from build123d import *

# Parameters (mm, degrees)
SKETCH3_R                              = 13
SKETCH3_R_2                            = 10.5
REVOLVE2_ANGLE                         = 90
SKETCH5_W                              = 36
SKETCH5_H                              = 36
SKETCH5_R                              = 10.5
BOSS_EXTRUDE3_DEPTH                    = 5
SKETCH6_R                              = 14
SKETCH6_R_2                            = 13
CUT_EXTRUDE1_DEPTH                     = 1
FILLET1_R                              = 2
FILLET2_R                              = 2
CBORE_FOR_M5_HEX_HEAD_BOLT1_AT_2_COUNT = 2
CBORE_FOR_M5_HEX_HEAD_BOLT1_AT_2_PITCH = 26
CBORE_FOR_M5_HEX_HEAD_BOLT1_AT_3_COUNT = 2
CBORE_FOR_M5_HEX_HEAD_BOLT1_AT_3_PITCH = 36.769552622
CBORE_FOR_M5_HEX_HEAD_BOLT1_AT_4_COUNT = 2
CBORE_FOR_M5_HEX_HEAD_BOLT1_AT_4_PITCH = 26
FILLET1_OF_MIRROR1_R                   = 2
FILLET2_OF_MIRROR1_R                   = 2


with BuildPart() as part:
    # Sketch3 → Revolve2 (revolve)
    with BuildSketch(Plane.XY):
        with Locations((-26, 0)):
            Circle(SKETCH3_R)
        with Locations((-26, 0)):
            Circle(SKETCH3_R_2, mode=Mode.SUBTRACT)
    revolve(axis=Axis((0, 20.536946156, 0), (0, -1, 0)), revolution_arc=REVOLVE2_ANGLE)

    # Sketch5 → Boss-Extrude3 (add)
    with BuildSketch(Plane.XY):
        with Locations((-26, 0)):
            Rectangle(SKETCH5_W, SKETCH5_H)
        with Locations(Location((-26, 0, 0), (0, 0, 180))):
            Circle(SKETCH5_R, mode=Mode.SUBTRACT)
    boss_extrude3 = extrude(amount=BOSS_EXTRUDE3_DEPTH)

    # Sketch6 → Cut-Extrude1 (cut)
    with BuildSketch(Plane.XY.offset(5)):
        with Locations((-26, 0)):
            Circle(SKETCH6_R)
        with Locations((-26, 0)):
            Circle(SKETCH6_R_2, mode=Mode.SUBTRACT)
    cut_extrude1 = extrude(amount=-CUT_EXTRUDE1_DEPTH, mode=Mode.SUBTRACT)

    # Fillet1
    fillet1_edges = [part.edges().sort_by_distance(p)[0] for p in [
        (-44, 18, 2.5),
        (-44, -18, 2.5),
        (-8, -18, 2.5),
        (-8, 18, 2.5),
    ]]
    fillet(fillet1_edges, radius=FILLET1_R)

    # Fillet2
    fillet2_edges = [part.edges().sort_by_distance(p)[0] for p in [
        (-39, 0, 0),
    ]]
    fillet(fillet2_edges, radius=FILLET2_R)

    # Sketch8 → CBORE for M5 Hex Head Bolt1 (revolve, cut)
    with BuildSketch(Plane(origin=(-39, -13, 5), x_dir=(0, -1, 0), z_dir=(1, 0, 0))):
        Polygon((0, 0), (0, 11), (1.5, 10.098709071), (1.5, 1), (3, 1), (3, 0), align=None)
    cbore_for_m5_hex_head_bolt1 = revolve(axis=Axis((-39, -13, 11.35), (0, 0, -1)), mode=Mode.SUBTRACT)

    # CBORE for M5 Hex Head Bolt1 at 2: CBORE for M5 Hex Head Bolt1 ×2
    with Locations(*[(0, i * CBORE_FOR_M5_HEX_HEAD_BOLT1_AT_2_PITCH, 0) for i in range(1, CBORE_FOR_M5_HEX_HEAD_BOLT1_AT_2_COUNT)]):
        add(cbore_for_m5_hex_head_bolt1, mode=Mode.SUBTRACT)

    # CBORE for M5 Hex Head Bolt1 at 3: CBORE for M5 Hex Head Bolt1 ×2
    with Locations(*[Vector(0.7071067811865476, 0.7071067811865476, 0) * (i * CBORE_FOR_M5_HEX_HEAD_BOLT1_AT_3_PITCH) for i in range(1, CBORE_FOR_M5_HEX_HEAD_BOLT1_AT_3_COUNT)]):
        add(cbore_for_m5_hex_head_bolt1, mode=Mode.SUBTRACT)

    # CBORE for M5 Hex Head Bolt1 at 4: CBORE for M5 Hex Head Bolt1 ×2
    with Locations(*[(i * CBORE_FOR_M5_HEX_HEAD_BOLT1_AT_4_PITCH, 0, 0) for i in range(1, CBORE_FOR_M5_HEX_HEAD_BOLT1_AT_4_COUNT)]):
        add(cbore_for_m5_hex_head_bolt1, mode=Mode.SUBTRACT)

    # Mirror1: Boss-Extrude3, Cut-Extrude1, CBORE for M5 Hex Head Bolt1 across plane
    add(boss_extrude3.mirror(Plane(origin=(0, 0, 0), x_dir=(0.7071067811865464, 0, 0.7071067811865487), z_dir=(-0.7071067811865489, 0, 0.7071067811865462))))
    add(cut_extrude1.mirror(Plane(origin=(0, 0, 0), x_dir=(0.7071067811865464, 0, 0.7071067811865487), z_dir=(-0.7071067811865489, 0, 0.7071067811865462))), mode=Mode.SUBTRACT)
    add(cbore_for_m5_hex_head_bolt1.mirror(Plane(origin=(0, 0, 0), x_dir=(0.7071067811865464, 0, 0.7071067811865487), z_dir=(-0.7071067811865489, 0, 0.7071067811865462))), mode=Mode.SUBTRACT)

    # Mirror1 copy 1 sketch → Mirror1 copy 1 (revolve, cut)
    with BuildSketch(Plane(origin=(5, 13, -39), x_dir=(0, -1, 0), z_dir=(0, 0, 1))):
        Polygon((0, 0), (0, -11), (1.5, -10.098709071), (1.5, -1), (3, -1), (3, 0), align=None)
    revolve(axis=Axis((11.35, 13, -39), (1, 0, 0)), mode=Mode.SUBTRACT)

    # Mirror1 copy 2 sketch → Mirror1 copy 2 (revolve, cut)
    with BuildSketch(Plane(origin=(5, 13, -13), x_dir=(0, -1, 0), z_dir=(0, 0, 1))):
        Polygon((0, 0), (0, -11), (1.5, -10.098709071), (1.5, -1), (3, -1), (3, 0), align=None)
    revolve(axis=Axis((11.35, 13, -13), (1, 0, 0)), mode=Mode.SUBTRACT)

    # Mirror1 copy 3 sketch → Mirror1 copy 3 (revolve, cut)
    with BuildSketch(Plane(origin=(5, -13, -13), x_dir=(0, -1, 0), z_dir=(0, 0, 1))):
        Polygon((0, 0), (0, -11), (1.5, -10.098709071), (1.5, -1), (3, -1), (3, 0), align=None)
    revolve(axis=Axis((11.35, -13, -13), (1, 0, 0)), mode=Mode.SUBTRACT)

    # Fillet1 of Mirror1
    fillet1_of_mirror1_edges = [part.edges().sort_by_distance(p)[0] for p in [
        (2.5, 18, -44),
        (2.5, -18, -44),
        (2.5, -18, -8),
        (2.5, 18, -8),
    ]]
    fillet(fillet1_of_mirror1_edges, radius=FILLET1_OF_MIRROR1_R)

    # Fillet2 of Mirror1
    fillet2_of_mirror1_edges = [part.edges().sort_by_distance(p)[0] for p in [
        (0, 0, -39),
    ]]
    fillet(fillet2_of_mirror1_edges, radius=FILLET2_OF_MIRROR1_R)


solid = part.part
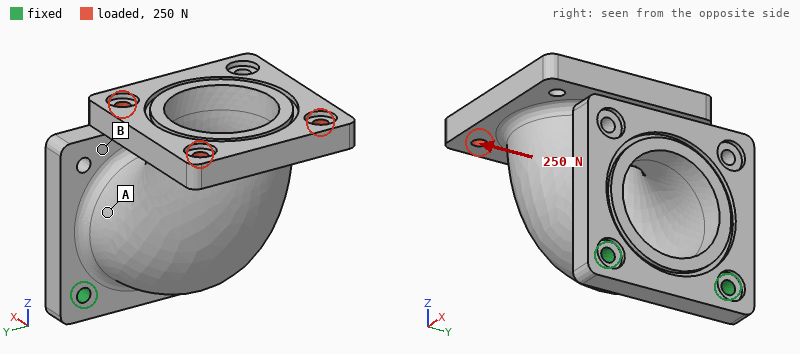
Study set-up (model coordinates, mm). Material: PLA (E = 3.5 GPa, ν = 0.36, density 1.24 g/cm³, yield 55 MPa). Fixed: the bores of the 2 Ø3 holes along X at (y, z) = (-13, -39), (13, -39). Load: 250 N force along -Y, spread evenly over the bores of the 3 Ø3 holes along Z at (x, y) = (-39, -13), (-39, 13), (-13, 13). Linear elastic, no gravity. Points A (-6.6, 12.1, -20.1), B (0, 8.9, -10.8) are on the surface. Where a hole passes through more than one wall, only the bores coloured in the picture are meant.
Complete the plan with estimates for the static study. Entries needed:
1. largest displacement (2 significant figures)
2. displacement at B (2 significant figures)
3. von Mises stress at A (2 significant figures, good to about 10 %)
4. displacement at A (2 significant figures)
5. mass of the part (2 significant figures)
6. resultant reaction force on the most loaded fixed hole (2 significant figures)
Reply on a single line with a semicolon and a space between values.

0.92 mm; 0.18 mm; 8.2 MPa; 0.22 mm; 20 g; 510 N
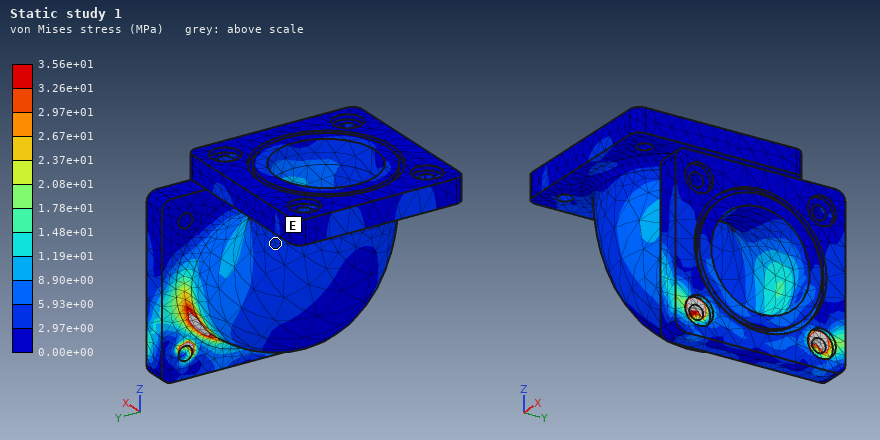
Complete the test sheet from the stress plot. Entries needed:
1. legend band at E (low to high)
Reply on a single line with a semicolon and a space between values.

2.97e+00 to 5.93e+00 MPa
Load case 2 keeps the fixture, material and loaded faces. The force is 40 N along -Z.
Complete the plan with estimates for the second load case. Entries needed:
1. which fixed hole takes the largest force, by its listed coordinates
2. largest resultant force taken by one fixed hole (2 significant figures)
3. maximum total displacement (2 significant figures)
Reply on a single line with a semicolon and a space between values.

(13, -39); 26 N; 0.79 mm
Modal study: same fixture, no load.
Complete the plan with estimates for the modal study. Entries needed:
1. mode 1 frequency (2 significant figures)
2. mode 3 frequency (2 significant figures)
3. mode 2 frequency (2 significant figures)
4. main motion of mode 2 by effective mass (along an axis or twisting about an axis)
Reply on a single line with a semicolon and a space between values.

330 Hz; 2000 Hz; 1000 Hz; along Y
